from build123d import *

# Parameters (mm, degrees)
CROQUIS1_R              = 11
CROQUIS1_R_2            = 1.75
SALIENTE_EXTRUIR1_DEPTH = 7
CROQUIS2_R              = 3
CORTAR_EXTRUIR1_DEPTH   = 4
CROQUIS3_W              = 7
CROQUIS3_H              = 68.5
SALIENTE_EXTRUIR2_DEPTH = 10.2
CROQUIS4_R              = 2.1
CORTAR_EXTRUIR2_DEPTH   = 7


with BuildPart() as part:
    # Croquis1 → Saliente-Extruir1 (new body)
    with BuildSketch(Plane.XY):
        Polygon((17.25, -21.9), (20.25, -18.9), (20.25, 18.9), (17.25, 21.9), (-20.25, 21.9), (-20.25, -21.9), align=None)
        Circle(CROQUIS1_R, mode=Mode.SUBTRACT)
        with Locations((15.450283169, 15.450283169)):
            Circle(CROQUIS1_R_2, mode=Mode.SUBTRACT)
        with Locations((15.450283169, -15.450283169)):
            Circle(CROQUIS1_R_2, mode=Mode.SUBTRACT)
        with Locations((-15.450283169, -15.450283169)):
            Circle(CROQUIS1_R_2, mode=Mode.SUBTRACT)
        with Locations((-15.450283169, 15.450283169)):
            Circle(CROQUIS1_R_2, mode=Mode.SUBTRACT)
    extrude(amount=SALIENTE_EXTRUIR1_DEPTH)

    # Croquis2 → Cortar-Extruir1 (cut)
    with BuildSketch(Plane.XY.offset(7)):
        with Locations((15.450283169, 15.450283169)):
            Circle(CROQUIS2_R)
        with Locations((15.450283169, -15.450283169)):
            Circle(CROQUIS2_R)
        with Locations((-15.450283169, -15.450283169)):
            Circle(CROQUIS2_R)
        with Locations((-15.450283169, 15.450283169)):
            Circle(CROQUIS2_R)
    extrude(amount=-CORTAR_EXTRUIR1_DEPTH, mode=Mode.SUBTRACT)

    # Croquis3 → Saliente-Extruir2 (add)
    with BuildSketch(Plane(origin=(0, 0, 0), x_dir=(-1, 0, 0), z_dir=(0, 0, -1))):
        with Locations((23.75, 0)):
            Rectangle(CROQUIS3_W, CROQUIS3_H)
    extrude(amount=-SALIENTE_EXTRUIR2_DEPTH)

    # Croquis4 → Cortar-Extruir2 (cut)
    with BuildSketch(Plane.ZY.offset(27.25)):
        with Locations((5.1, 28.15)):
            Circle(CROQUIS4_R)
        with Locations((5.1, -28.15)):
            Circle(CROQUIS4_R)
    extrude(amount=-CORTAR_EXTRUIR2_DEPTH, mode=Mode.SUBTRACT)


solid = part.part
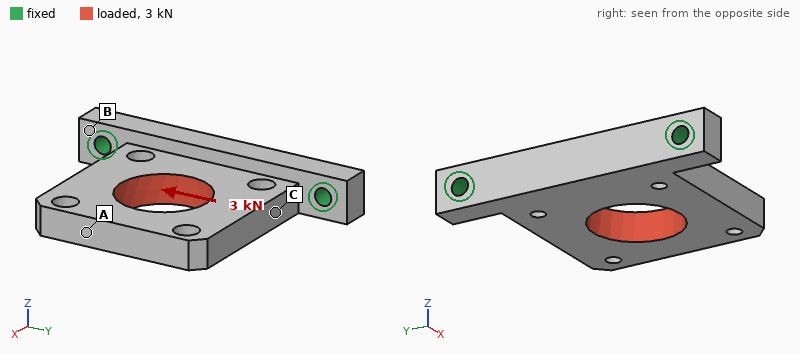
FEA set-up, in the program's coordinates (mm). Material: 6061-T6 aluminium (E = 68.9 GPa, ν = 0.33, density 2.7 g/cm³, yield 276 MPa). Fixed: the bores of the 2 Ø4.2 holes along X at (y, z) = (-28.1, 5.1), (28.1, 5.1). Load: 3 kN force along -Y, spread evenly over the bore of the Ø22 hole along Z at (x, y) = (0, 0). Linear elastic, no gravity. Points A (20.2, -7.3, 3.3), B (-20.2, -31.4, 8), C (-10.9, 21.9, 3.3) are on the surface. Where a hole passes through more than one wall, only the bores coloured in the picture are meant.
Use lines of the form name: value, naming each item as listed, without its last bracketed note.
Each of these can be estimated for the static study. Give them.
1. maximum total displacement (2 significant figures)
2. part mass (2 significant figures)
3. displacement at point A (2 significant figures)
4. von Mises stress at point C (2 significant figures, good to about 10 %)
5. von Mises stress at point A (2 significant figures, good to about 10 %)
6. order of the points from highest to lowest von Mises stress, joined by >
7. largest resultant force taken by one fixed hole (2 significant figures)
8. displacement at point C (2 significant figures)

maximum total displacement: 67 µm
part mass: 37 g
displacement at point A: 62 µm
von Mises stress at point C: 36 MPa
von Mises stress at point A: 18 MPa
order of the points from highest to lowest von Mises stress, joined by >: C > A > B
largest resultant force taken by one fixed hole: 2.1 kN
displacement at point C: 25 µm
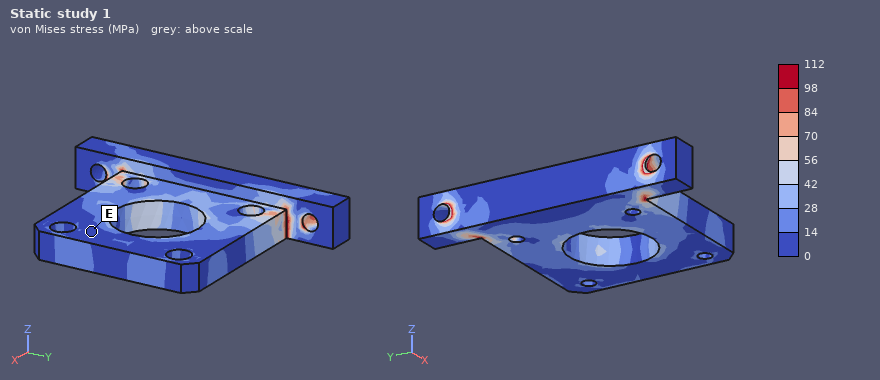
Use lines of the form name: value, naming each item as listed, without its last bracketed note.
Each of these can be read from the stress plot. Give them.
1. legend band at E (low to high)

legend band at E: 0 to 14 MPa
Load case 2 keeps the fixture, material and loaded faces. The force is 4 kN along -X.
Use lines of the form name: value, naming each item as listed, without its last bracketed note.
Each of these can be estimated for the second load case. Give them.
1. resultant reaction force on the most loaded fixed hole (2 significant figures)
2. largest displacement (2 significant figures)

resultant reaction force on the most loaded fixed hole: 2.2 kN
largest displacement: 60 µm
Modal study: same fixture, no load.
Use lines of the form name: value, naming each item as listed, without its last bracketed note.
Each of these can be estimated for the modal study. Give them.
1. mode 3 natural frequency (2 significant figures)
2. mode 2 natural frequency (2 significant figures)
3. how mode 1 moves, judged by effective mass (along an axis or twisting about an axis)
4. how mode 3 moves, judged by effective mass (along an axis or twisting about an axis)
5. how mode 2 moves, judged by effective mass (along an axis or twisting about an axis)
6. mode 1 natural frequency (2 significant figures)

mode 3 natural frequency: 7700 Hz
mode 2 natural frequency: 5400 Hz
how mode 1 moves, judged by effective mass: along Z
how mode 3 moves, judged by effective mass: along Y
how mode 2 moves, judged by effective mass: twisting about X
mode 1 natural frequency: 1800 Hz
